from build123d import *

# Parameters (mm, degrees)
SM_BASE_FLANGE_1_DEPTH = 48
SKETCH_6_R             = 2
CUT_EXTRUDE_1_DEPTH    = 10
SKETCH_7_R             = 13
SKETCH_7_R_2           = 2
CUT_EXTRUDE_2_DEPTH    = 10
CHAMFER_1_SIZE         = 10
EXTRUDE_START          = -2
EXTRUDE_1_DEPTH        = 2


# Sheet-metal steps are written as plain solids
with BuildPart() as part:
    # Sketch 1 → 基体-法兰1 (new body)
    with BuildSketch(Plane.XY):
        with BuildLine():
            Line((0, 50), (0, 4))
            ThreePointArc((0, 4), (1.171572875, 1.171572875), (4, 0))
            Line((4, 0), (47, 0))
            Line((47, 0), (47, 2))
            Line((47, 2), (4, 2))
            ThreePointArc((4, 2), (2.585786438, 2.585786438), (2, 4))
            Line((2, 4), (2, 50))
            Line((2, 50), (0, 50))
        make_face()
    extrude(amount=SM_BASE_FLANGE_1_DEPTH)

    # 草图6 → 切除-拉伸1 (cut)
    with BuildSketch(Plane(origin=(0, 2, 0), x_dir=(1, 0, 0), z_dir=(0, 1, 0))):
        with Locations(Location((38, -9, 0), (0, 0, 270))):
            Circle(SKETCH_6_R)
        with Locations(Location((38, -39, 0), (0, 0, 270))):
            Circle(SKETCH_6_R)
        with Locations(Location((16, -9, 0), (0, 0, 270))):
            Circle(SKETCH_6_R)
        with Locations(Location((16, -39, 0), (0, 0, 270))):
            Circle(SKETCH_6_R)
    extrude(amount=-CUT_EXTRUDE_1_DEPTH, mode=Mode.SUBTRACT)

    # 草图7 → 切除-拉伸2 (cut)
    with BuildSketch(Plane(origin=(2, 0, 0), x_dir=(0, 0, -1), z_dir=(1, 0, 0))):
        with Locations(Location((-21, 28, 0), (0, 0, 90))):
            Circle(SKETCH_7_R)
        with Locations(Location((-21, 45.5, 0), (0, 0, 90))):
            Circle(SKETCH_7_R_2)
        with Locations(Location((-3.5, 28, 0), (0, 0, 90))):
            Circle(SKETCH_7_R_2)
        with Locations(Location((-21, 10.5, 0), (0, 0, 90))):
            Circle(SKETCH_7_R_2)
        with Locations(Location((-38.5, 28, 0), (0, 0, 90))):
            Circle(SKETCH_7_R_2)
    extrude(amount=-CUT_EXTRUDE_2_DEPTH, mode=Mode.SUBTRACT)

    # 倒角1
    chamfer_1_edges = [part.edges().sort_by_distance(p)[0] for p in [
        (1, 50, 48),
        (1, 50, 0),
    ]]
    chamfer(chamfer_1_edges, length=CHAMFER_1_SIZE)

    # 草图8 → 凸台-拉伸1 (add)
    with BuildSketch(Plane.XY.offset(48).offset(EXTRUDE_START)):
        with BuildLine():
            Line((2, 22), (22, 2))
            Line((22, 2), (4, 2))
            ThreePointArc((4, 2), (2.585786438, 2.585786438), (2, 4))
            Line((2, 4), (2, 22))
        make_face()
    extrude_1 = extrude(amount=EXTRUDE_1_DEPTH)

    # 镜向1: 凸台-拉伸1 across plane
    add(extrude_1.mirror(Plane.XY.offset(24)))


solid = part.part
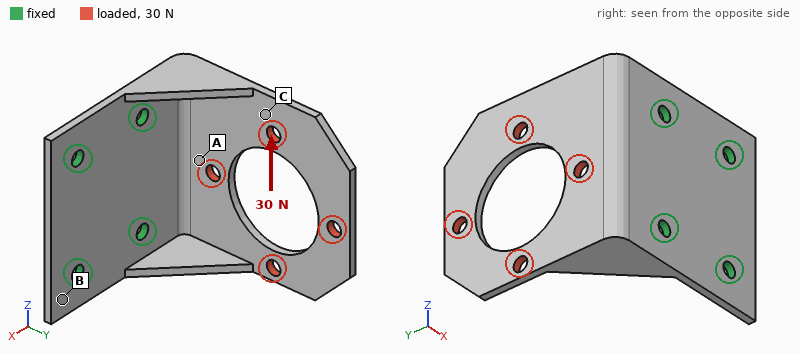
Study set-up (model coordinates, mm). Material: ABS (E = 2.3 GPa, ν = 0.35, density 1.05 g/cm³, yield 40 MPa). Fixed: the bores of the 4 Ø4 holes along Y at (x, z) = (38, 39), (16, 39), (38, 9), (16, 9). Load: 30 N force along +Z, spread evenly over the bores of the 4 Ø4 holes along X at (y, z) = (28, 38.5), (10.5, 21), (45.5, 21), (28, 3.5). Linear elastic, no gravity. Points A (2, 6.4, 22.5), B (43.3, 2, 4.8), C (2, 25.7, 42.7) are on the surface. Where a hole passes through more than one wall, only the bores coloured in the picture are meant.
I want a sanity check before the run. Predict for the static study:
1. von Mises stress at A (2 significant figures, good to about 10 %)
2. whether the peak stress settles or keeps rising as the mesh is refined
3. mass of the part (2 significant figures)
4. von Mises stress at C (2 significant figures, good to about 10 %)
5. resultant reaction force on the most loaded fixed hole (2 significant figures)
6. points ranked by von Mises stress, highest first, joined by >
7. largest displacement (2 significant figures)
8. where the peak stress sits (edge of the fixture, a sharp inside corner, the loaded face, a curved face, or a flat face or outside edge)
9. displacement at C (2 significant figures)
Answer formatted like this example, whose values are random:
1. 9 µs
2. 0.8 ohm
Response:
1. 5.0 MPa
2. keeps rising
3. 8.7 g
4. 2.9 MPa
5. 33 N
6. A > C > B
7. 0.98 mm
8. edge of the fixture
9. 0.63 mm
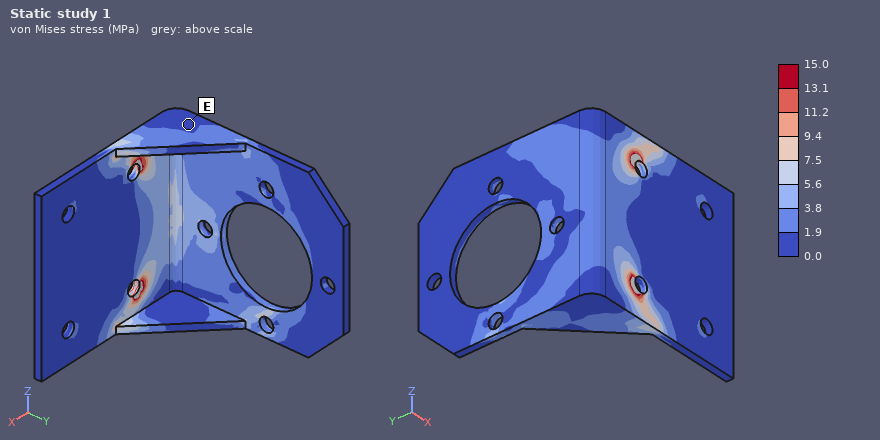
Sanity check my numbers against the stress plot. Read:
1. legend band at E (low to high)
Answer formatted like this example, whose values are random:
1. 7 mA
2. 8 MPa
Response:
1. 0.0 to 1.9 MPa
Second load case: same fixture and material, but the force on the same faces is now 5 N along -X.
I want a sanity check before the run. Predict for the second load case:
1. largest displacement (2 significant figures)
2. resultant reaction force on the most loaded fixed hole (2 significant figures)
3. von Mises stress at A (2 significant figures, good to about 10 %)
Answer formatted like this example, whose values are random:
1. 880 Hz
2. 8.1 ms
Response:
1. 0.90 mm
2. 3.2 N
3. 0.47 MPa
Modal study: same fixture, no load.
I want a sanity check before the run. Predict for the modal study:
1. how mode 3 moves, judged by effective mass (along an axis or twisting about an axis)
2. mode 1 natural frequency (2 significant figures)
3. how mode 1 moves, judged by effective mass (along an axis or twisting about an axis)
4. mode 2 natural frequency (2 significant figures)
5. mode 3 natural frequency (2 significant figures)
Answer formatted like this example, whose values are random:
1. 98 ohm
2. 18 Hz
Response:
1. along Y
2. 280 Hz
3. along X
4. 500 Hz
5. 830 Hz
